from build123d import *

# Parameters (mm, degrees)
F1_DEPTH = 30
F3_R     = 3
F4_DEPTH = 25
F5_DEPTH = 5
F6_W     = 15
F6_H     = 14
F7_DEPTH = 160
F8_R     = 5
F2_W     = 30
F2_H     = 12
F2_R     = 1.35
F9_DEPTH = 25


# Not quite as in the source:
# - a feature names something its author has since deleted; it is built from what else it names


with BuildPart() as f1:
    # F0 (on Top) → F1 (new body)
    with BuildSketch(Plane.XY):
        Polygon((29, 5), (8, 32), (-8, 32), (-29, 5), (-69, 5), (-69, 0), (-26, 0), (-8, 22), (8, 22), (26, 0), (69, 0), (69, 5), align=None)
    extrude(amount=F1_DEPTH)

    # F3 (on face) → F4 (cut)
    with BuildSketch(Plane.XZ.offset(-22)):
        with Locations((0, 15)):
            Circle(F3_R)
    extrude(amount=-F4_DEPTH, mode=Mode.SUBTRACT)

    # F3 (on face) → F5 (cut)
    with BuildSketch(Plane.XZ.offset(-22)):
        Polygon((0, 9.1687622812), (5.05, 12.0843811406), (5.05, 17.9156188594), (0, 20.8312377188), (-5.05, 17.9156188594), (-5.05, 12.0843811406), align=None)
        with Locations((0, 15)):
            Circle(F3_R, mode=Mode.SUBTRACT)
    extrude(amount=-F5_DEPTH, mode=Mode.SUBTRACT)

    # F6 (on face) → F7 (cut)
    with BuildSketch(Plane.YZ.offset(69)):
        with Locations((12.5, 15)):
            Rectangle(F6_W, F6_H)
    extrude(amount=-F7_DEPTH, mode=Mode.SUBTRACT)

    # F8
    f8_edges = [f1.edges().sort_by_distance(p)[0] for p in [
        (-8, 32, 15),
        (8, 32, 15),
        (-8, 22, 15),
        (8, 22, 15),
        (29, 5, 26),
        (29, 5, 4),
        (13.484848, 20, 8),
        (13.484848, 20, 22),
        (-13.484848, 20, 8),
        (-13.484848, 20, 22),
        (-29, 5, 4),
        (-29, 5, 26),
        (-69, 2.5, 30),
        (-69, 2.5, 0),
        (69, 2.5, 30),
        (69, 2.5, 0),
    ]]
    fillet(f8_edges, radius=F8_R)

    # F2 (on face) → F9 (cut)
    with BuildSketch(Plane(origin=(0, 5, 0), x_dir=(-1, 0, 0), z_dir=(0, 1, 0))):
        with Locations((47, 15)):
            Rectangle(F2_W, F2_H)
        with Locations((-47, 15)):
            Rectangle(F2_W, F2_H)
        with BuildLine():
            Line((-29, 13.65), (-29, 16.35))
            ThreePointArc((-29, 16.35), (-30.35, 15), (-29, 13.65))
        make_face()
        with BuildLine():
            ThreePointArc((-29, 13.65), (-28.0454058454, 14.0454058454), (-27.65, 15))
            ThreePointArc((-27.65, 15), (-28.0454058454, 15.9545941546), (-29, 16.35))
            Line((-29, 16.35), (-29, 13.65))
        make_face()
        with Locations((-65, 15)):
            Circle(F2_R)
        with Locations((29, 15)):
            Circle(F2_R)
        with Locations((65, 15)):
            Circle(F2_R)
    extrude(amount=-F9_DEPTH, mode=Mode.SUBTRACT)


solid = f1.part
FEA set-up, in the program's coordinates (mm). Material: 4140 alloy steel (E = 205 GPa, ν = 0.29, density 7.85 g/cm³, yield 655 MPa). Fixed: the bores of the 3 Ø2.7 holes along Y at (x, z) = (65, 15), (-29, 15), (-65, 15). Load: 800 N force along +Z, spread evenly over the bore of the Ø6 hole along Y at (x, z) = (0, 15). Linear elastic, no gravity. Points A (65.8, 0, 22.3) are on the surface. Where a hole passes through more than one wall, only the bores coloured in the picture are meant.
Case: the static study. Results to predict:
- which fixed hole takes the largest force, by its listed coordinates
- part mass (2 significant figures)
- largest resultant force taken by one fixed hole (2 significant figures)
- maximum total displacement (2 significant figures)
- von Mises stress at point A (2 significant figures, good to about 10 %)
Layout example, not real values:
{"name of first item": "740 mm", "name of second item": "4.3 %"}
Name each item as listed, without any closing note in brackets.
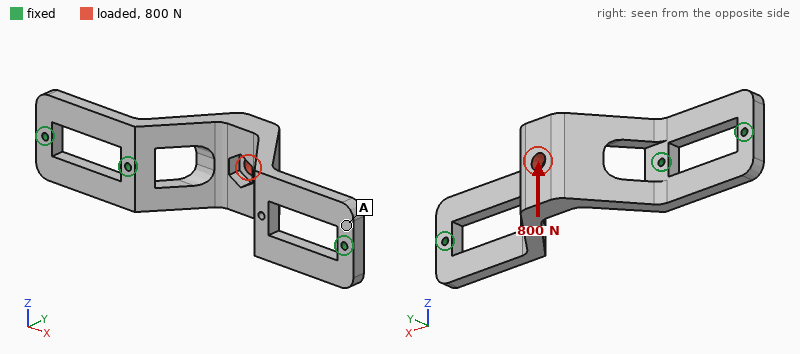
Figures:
{"which fixed hole takes the largest force, by its listed coordinates": "(-29, 15)", "part mass": "160 g", "largest resultant force taken by one fixed hole": "990 N", "maximum total displacement": "0.10 mm", "von Mises stress at point A": "40 MPa"}
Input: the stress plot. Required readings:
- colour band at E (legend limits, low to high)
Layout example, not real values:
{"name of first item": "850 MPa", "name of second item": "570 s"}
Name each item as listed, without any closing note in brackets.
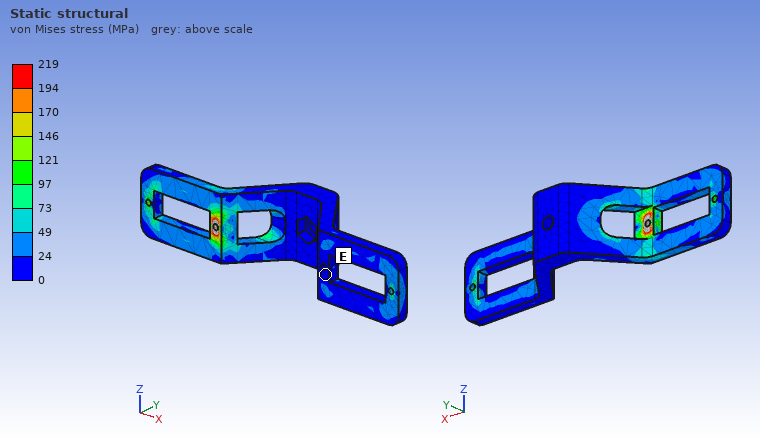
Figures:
{"colour band at E": "0 to 24 MPa"}
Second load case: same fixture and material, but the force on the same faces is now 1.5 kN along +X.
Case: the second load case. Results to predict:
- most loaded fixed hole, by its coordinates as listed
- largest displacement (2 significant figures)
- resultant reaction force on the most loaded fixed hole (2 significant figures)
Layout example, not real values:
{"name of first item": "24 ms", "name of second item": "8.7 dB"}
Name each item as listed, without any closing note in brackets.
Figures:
{"most loaded fixed hole, by its coordinates as listed": "(65, 15)", "largest displacement": "93 µm", "resultant reaction force on the most loaded fixed hole": "990 N"}
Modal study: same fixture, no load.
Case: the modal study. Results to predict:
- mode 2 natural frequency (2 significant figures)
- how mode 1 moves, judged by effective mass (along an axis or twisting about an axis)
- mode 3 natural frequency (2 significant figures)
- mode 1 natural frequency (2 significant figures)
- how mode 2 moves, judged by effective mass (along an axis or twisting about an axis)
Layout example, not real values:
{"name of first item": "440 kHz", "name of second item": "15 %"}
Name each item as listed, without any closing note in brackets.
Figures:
{"mode 2 natural frequency": "1900 Hz", "how mode 1 moves, judged by effective mass": "along Y", "mode 3 natural frequency": "3400 Hz", "mode 1 natural frequency": "1800 Hz", "how mode 2 moves, judged by effective mass": "along Z"}
